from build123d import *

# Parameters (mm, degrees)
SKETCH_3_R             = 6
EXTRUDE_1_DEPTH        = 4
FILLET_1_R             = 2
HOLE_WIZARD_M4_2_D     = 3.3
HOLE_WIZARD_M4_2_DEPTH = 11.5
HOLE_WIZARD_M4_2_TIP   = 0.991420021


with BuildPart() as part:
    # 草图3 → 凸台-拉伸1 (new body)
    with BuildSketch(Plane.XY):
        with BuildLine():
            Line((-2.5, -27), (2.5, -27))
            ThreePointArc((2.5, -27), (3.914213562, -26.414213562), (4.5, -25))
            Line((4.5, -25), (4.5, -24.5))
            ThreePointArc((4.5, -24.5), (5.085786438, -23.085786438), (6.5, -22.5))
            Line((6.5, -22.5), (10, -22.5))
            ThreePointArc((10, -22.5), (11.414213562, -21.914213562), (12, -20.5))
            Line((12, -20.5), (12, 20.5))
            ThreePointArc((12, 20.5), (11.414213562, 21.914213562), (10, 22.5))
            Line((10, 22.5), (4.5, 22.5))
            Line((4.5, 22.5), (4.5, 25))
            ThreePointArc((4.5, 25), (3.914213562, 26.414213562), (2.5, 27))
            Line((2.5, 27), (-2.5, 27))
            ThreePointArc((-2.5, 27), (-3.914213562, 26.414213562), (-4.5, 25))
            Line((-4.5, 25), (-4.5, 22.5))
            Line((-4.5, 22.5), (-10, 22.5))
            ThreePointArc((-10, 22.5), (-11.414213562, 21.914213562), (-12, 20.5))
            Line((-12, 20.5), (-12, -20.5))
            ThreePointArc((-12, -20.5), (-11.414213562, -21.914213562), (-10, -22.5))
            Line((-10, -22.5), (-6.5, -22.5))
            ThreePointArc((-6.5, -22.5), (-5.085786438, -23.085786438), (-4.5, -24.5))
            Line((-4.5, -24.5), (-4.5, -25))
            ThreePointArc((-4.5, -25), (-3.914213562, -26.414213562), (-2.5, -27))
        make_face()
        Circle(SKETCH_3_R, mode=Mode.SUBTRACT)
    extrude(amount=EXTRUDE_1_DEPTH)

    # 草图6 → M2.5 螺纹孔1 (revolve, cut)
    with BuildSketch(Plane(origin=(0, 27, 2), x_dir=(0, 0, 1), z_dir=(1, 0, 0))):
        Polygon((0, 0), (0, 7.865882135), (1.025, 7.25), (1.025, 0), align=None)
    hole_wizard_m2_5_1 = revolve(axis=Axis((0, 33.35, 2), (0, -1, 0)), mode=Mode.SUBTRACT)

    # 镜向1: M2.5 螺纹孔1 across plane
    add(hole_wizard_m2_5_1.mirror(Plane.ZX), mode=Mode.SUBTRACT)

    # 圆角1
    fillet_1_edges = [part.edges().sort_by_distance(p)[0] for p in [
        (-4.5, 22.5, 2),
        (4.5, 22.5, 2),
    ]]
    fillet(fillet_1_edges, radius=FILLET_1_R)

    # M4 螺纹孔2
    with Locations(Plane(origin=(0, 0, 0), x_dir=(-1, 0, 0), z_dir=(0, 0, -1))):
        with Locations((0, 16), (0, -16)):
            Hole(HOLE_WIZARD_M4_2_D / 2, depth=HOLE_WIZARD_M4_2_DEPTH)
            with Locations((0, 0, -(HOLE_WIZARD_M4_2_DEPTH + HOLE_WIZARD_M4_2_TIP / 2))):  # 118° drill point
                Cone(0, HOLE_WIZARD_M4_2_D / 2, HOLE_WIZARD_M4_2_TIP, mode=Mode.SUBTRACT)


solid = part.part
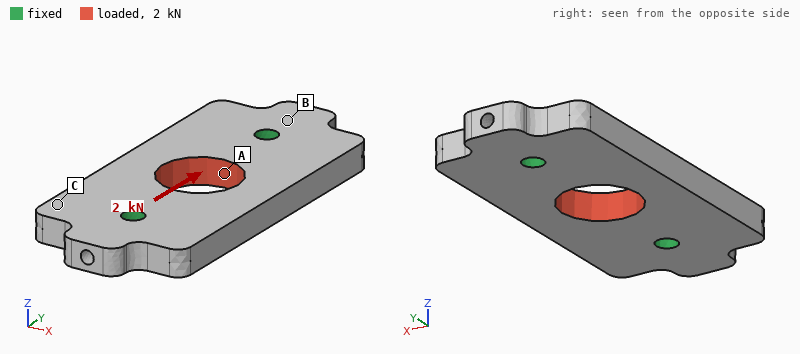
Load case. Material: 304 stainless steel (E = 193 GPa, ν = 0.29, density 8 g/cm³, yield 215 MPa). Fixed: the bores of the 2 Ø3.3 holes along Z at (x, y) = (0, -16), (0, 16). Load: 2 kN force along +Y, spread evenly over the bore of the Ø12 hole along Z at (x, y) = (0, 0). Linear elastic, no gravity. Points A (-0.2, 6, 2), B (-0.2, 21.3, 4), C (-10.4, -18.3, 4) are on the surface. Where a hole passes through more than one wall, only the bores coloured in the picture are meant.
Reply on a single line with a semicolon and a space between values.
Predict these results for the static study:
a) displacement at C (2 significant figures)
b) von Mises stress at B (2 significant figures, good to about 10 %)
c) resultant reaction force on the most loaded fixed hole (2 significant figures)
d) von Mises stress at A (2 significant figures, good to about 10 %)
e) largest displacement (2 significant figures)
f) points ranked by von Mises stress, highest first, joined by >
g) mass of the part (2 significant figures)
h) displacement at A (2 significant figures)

0.83 µm; 11 MPa; 1.0 kN; 20 MPa; 1.5 µm; A > B > C; 32 g; 0.96 µm
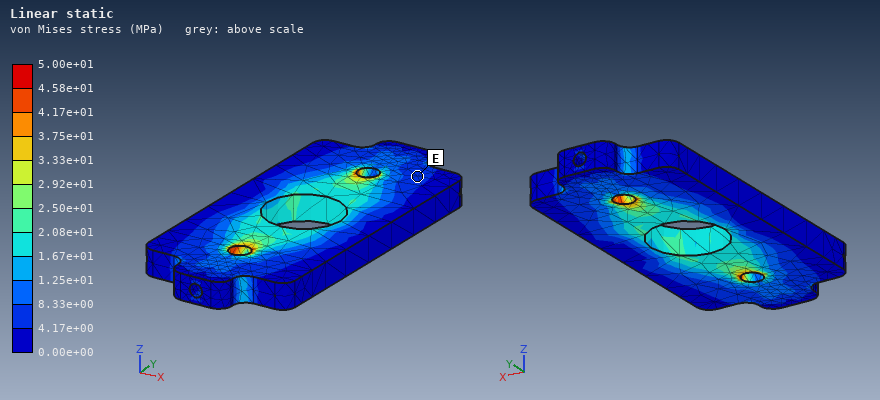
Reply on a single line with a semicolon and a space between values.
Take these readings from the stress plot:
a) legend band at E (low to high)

4.17e+00 to 8.33e+00 MPa
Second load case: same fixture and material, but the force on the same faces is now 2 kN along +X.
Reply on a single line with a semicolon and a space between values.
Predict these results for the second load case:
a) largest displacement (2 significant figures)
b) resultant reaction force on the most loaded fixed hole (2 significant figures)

3.7 µm; 1.0 kN
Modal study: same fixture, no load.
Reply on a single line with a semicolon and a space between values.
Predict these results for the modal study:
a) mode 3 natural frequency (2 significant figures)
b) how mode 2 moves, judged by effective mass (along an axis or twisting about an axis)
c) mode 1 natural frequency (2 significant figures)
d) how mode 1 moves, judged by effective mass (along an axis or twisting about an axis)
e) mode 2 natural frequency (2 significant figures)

21 kHz; along Z; 13 kHz; twisting about Y; 15 kHz
